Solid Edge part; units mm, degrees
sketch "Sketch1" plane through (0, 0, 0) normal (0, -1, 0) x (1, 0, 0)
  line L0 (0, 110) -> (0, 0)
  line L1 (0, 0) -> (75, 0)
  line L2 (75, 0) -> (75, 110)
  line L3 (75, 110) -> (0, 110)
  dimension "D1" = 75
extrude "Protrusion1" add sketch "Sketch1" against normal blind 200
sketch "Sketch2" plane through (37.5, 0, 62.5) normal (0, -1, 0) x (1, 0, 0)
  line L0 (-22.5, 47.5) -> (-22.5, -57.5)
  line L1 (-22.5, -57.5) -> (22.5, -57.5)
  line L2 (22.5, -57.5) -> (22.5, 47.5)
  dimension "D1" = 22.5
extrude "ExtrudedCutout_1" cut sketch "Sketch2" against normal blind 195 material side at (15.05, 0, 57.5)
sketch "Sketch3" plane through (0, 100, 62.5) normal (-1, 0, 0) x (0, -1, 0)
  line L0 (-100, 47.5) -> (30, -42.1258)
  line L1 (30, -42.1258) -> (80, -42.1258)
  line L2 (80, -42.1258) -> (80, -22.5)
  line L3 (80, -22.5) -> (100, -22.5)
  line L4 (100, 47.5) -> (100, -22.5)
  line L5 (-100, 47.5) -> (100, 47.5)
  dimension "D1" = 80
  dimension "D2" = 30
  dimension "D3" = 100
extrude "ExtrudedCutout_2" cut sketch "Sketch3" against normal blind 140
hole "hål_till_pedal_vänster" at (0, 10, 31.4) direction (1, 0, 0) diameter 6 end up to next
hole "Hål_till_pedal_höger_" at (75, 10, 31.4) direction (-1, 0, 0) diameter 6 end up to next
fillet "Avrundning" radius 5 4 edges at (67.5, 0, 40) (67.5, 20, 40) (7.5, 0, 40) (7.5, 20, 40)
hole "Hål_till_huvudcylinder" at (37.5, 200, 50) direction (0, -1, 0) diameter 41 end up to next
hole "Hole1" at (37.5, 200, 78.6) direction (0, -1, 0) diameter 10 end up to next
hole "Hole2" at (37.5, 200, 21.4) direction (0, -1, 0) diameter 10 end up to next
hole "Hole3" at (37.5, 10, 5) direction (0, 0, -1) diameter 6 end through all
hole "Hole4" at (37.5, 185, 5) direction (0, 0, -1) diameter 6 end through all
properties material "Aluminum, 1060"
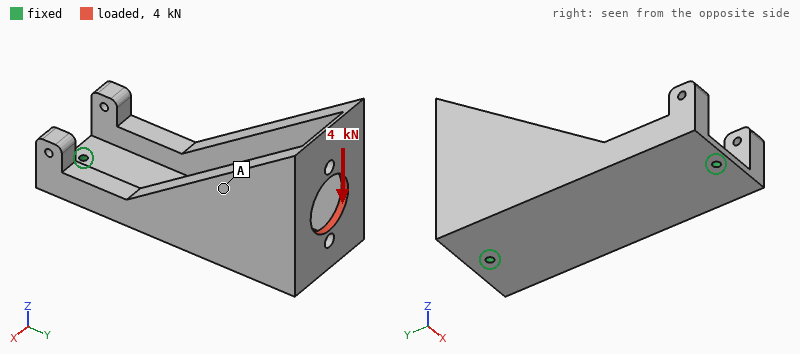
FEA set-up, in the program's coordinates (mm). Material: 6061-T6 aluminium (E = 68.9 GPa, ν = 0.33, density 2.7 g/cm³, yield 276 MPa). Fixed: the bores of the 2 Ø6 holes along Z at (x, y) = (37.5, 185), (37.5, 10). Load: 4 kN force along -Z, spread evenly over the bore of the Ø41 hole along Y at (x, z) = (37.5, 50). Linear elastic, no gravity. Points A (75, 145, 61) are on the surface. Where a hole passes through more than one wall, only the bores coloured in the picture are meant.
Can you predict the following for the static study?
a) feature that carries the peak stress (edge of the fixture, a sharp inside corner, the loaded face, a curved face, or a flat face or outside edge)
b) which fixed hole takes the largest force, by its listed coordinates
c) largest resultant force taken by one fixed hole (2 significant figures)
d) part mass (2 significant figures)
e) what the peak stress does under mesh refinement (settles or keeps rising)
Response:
edge of the fixture
(37.5, 185)
4.2 kN
990 g
keeps rising
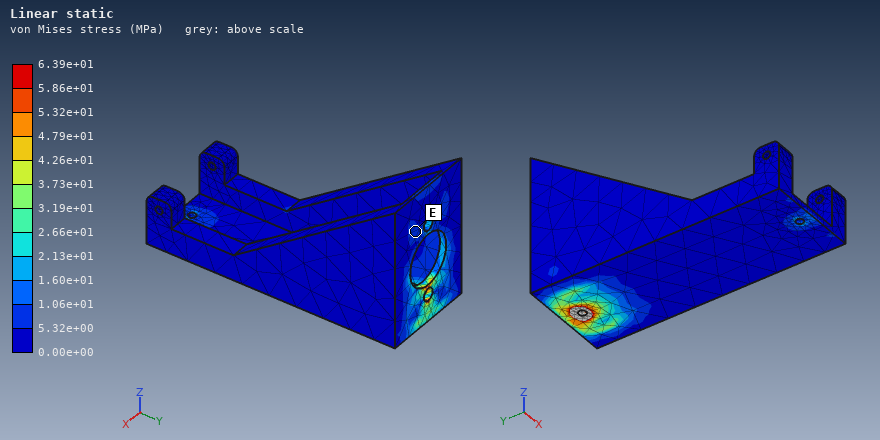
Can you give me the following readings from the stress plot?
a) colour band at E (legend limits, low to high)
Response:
5.32e+00 to 1.06e+01 MPa
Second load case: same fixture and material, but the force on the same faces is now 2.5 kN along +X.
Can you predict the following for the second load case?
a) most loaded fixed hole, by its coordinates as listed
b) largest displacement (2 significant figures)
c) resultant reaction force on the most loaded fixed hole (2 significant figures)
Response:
(37.5, 185)
1.7 mm
2.6 kN
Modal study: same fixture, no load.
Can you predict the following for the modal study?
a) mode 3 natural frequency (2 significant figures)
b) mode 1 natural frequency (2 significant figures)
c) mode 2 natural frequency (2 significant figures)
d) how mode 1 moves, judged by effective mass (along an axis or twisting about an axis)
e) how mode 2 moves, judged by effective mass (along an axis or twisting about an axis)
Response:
1500 Hz
310 Hz
1100 Hz
along X
along Z
